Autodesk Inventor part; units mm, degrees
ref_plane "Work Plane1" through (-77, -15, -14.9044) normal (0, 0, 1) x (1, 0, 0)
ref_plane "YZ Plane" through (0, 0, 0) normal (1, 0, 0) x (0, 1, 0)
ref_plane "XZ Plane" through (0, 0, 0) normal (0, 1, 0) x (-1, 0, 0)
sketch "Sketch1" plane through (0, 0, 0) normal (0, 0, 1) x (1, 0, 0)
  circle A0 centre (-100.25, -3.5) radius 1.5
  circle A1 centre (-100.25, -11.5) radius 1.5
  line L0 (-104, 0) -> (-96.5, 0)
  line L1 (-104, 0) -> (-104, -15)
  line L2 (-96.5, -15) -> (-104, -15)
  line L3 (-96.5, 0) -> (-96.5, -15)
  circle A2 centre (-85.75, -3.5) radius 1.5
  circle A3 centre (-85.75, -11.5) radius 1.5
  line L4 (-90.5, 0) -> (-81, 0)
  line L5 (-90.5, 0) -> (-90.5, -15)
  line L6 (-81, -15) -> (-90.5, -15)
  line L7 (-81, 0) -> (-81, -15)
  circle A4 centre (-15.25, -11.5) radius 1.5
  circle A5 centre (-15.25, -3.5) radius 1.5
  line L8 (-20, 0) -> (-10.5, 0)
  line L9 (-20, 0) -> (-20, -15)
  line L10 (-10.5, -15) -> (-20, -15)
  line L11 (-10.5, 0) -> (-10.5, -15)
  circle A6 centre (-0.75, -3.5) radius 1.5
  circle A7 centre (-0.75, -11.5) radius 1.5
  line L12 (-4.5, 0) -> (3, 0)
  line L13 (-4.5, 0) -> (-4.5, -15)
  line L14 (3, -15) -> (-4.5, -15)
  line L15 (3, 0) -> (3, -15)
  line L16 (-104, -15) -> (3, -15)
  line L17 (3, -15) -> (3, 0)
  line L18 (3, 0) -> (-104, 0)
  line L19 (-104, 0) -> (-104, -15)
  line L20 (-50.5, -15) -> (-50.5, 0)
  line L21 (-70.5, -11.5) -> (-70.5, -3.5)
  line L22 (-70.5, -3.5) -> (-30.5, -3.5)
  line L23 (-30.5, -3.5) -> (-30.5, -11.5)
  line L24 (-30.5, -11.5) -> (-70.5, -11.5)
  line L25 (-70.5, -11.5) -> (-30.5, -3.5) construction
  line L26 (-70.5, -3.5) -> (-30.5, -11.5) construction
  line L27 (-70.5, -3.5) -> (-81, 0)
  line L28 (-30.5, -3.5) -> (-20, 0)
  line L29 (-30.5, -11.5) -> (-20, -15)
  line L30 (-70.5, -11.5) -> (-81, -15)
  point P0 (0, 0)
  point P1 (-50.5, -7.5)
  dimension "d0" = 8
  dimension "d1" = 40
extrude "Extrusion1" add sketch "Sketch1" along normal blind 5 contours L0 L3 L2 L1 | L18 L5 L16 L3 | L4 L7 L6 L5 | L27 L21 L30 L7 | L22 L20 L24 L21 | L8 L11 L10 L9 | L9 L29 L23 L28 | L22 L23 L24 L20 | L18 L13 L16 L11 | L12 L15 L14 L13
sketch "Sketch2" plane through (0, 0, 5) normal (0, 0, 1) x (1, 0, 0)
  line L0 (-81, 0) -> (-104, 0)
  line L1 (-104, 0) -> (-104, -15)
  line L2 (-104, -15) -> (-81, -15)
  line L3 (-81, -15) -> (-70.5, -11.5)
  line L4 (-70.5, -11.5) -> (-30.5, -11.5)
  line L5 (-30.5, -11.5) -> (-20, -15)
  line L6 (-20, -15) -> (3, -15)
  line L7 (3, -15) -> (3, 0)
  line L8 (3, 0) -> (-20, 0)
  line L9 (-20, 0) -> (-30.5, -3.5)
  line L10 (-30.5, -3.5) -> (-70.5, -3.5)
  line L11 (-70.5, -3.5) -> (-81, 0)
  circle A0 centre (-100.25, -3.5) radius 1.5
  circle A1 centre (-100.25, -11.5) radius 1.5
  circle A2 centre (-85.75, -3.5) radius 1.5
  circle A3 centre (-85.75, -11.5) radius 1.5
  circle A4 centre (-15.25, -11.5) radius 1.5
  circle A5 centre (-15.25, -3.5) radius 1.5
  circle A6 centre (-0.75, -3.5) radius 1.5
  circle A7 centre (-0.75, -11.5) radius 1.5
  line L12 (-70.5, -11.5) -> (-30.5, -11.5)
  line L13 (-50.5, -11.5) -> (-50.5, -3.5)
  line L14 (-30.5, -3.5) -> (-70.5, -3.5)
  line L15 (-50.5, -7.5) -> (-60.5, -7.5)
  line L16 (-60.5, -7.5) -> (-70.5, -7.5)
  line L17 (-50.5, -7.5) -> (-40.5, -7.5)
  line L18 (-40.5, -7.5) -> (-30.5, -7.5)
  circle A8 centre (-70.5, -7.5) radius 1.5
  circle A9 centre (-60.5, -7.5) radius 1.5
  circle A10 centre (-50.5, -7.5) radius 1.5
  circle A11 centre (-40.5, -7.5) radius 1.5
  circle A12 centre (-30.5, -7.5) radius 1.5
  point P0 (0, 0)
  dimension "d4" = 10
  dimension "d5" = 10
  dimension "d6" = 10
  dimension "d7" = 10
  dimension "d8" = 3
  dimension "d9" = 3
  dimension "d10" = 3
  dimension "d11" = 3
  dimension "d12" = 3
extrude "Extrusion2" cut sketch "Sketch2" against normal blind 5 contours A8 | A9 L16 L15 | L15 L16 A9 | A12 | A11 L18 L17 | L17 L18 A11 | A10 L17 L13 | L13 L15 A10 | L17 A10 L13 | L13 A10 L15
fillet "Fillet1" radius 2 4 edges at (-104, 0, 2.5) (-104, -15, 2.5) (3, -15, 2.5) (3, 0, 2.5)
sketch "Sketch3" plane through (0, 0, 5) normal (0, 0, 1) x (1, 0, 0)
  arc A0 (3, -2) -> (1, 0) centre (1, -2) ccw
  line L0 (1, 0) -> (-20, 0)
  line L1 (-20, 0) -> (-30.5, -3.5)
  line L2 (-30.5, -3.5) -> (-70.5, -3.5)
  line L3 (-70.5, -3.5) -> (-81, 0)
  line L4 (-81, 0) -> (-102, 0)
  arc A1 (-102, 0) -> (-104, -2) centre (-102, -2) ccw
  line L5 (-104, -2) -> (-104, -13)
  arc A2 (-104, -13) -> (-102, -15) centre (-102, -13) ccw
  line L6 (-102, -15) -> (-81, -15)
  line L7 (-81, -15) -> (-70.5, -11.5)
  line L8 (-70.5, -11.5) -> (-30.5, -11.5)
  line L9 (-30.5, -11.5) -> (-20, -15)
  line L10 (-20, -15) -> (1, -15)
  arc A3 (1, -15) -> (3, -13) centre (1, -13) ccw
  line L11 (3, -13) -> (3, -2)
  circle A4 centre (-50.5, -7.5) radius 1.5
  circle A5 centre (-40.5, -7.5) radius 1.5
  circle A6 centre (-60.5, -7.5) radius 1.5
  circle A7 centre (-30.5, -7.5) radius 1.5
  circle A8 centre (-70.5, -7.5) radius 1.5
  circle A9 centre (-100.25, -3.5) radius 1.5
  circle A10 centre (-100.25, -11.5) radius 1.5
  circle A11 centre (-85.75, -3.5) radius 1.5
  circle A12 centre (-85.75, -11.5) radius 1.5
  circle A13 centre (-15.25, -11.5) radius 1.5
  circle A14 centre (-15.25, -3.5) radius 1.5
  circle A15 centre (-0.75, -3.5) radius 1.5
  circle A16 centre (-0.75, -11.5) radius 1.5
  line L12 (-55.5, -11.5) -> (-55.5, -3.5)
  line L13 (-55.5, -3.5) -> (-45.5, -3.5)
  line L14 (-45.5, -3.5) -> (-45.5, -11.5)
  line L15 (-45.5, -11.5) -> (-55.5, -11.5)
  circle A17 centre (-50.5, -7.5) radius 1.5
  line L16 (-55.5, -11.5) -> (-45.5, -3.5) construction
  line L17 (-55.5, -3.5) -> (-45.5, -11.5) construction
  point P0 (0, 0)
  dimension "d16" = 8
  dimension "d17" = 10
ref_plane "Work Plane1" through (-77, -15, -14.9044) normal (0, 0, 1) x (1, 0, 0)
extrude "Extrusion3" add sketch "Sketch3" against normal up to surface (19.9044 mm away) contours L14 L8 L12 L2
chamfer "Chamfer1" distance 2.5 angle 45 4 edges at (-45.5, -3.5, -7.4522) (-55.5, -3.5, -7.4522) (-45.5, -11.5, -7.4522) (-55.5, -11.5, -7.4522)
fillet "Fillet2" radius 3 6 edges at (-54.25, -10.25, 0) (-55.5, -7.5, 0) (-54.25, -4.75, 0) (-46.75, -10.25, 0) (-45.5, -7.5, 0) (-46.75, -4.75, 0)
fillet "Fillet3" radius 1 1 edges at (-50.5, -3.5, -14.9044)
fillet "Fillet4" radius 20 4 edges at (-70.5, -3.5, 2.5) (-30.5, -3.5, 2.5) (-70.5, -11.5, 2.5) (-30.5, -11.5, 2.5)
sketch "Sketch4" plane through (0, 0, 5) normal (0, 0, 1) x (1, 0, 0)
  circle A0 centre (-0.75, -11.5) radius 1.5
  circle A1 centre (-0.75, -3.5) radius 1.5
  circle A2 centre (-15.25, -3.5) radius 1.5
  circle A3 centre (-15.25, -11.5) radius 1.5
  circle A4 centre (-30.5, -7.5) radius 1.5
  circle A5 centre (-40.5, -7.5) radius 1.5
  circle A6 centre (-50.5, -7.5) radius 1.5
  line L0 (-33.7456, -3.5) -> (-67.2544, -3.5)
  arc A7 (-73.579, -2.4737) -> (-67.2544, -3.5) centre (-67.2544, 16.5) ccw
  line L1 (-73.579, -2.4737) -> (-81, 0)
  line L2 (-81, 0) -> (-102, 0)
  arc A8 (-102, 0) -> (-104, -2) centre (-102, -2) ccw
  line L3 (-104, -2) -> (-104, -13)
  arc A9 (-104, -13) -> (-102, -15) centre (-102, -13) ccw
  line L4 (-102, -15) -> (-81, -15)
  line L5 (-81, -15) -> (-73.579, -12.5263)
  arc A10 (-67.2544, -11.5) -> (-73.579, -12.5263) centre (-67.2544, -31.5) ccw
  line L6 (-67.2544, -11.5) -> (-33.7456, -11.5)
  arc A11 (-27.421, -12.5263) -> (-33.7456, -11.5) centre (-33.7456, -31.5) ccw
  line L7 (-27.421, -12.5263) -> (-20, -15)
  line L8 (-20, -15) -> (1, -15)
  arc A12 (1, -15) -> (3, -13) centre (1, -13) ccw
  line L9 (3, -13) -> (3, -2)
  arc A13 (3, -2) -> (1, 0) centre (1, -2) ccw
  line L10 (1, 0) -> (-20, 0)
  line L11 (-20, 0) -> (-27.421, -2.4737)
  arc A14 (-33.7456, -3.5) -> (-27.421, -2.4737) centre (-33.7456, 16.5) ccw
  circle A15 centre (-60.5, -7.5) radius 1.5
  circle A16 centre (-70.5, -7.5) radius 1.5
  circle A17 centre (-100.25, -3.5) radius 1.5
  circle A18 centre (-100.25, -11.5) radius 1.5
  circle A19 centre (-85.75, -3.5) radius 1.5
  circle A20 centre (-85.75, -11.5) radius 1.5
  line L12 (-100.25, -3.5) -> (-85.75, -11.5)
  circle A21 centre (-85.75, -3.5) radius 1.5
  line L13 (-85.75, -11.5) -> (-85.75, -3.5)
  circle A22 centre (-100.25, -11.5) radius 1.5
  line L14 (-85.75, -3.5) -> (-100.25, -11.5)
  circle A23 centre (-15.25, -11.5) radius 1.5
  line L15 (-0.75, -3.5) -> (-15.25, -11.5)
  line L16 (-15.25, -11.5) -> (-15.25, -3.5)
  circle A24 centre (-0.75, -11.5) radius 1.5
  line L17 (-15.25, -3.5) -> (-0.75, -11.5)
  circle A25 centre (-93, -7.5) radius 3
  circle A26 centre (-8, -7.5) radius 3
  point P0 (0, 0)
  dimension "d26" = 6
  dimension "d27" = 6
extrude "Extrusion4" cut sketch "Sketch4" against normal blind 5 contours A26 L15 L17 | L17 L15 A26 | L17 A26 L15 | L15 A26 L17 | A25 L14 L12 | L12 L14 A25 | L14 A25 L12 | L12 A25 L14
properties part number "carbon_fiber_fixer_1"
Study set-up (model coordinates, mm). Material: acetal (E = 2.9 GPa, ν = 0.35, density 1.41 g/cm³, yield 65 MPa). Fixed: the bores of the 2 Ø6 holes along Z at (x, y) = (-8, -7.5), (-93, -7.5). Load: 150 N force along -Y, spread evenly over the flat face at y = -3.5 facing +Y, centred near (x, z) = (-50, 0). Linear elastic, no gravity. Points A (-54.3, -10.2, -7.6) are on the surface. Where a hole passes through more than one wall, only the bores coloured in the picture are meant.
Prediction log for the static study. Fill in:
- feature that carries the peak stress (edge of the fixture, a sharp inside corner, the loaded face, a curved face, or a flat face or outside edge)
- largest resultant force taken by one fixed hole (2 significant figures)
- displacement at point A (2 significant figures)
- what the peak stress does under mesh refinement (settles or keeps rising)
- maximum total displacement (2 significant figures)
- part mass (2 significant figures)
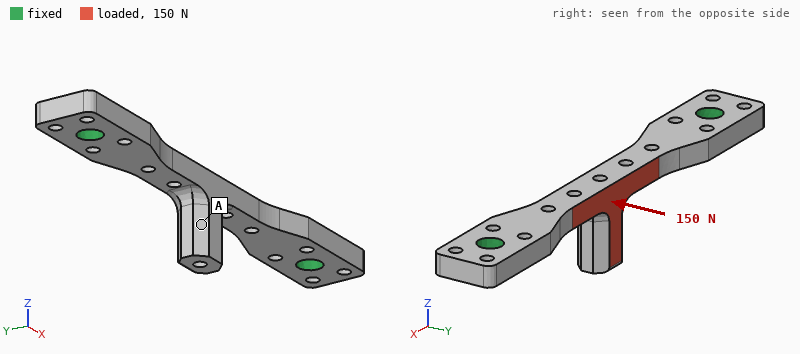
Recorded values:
a sharp inside corner
75 N
0.70 mm
keeps rising
0.95 mm
9.1 g
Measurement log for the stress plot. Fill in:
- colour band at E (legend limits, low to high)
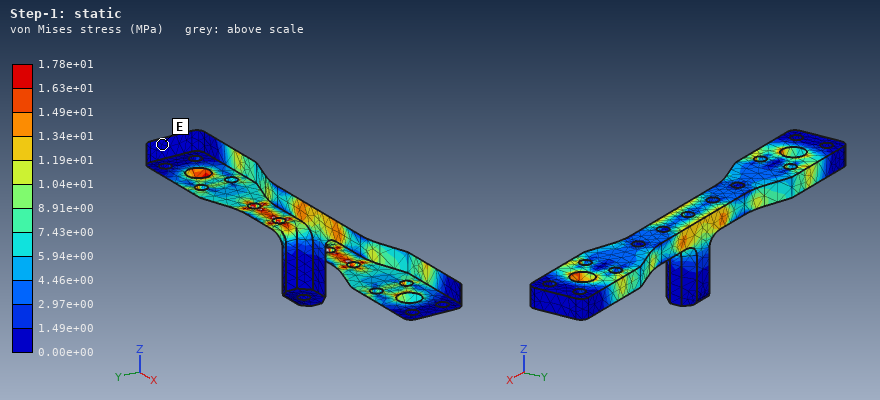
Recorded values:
0.00e+00 to 1.49e+00 MPa
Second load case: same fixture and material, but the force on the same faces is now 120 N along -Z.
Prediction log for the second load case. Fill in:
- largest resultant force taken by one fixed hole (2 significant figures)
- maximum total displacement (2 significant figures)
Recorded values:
63 N
1.2 mm
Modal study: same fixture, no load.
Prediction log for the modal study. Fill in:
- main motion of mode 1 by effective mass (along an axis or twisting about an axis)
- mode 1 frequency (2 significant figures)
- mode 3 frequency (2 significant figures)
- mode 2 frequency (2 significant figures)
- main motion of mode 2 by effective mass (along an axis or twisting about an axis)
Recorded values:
along Z
1000 Hz
2200 Hz
1200 Hz
along Y
